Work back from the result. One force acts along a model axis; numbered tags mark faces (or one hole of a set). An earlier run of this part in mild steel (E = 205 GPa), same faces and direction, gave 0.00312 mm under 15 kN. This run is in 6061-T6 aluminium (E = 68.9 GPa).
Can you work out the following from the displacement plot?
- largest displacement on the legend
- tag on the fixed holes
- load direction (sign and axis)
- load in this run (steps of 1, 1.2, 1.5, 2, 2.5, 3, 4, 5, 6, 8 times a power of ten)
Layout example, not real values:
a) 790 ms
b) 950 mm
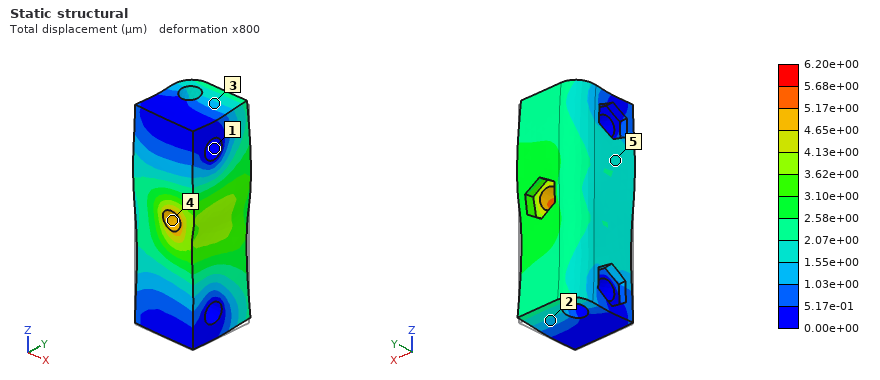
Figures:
a) 6.20e+00 µm
b) 1
c) +Z
d) 10 kN
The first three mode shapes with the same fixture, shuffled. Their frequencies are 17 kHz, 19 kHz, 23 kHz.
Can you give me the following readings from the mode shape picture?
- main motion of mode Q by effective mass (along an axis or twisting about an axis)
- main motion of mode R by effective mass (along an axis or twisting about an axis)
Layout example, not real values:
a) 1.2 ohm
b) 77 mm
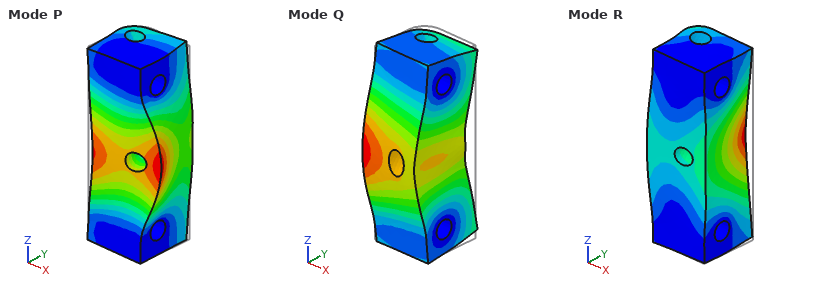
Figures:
a) along Y
b) along X
